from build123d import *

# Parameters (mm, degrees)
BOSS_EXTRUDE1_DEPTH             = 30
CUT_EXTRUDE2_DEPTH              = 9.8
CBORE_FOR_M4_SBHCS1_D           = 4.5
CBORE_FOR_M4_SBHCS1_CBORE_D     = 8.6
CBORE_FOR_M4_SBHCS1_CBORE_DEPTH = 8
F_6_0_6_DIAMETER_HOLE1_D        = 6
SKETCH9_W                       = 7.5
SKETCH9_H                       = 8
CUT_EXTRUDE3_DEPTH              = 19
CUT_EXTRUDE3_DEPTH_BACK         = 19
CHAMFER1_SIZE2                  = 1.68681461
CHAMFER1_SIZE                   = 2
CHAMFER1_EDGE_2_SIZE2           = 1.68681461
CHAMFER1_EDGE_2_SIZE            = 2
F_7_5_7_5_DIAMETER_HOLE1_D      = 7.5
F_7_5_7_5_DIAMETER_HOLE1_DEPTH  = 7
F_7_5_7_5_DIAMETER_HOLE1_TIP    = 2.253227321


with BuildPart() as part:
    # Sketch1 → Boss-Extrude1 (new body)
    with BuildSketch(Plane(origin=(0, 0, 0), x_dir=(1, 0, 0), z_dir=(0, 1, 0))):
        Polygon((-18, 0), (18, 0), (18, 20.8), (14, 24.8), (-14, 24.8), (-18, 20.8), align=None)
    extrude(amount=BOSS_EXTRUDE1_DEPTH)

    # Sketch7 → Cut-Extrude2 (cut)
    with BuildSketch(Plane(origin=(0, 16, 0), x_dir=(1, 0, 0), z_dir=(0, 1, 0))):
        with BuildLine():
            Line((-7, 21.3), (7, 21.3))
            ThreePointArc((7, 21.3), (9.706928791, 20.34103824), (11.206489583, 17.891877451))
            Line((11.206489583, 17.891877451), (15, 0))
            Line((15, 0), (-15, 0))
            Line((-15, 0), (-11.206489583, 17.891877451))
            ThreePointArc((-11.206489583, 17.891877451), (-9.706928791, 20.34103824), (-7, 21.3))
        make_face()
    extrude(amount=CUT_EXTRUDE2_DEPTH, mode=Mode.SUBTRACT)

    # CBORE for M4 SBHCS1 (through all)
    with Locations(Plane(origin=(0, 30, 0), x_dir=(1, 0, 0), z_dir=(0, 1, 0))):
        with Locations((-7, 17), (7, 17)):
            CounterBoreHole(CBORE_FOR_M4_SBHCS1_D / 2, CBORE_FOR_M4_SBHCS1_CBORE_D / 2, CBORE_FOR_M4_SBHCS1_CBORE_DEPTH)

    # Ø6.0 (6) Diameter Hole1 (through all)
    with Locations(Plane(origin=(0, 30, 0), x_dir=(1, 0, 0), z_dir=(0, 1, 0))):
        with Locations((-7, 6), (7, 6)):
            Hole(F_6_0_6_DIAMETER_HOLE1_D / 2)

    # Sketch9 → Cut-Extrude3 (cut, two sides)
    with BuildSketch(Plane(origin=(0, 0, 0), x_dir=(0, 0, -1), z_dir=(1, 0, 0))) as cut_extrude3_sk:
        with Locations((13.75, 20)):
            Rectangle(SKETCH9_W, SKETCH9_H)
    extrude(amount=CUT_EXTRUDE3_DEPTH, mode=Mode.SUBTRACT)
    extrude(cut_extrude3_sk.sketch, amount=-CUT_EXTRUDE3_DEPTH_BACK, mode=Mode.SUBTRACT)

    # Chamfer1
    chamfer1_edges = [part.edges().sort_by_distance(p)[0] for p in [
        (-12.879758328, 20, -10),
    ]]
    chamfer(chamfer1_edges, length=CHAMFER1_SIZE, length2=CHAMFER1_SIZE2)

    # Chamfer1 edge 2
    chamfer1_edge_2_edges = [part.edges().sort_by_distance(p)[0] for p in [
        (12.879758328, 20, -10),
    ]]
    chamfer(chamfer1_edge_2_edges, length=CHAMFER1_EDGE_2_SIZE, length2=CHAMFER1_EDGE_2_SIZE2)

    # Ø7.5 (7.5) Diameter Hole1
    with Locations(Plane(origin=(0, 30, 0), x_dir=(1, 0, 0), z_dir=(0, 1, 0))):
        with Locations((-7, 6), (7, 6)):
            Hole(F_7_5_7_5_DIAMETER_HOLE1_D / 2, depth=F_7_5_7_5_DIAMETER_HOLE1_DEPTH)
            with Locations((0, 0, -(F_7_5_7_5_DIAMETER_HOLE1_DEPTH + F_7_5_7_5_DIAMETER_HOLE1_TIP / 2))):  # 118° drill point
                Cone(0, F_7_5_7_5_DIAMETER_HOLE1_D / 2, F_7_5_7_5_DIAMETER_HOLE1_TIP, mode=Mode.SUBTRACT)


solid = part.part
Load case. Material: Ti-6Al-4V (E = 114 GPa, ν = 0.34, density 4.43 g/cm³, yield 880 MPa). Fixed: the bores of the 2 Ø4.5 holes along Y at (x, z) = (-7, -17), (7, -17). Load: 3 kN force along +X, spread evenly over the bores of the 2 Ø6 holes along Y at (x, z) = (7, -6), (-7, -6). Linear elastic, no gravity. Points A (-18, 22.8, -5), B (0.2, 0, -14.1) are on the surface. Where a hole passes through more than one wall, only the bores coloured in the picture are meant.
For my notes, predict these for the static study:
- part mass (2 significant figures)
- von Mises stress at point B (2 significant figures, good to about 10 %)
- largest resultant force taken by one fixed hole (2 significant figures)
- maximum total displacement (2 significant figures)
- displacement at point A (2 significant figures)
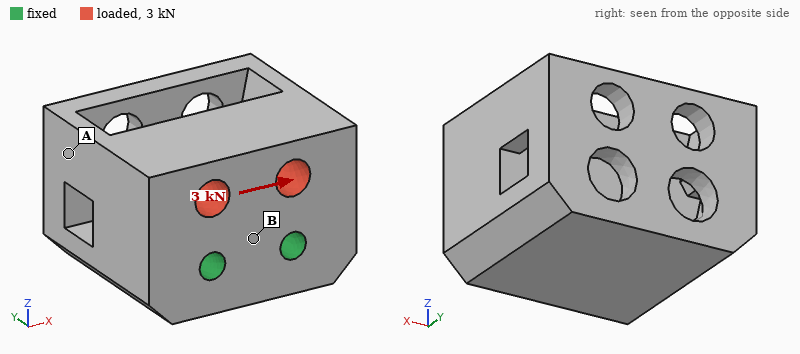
80 g
10 MPa
2.2 kN
4.4 µm
3.0 µm
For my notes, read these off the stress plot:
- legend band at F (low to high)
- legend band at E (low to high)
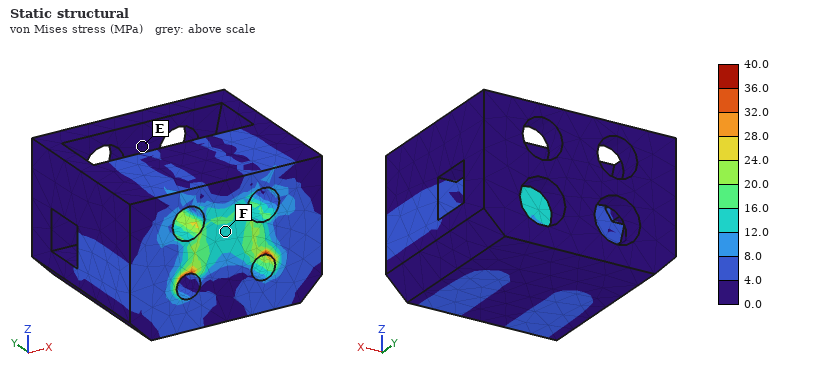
12.0 to 16.0 MPa
0.0 to 4.0 MPa
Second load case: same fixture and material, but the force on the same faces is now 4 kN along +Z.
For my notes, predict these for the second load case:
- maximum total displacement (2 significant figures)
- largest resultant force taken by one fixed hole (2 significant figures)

1.8 µm
2.0 kN
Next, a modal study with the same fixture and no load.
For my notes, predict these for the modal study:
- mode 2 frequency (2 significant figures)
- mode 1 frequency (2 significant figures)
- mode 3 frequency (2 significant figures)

13 kHz
12 kHz
18 kHz
